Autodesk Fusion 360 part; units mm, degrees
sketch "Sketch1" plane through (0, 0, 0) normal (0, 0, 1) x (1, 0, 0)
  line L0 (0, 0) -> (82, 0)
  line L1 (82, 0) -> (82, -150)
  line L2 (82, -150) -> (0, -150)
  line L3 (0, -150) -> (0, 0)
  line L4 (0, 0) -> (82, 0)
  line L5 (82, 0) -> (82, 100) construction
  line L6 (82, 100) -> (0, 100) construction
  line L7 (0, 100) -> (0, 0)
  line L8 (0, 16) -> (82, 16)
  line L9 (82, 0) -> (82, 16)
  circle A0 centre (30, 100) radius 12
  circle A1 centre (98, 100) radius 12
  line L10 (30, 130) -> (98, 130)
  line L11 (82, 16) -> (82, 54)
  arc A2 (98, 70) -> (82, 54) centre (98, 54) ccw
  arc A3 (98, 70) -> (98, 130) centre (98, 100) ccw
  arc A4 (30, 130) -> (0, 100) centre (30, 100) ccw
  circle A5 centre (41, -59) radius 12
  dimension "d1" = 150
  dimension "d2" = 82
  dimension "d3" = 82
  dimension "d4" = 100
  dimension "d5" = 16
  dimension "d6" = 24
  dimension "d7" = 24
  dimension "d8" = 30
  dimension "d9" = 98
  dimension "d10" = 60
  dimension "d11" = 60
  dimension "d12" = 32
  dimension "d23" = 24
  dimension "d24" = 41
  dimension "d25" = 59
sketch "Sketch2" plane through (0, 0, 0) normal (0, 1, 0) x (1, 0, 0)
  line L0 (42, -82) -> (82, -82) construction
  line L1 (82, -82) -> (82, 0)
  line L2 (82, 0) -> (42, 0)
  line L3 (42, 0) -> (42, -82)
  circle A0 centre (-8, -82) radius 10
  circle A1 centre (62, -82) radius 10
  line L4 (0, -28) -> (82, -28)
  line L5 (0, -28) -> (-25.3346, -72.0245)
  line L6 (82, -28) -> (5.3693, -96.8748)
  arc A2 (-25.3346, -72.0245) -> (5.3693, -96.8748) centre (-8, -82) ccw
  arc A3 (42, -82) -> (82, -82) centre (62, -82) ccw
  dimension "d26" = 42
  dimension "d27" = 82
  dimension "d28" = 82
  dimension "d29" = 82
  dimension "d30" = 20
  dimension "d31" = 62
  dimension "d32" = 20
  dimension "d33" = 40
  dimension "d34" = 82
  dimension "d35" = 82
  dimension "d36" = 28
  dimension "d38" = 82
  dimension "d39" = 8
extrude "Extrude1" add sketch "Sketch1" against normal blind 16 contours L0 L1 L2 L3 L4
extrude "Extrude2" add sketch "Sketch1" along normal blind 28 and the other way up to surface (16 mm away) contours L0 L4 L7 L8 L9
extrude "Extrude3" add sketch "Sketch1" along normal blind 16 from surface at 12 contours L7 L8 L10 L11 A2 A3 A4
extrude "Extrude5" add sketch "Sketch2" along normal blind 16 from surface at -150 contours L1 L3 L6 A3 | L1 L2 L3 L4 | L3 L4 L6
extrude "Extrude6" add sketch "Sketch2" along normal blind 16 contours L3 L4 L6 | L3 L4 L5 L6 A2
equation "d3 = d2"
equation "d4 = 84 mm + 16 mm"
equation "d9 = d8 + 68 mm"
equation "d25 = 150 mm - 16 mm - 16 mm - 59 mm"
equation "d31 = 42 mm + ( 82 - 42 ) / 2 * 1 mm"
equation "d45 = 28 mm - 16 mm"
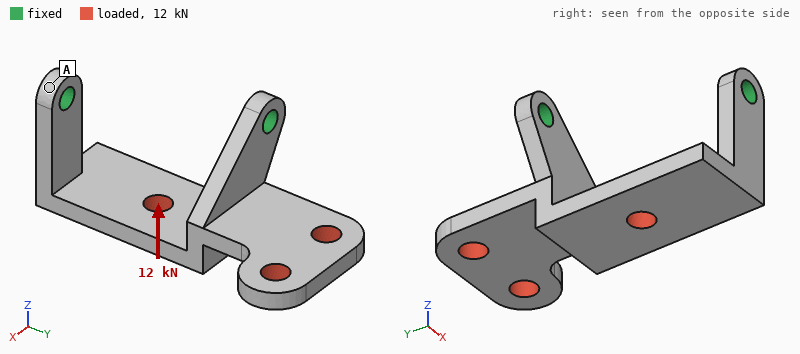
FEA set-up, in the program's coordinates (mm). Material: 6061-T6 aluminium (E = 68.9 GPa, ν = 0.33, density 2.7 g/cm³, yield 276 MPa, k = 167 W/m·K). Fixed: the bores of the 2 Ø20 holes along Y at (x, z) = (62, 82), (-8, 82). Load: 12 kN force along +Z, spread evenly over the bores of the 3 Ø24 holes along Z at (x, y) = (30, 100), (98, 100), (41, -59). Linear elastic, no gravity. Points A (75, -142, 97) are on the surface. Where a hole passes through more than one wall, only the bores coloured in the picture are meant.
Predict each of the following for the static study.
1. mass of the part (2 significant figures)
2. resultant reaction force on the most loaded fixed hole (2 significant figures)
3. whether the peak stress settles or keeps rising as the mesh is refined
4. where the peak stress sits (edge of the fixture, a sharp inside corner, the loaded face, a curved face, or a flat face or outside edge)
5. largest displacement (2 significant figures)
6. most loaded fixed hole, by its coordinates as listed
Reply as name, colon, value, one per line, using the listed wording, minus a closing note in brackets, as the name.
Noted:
mass of the part: 1.5 kg
resultant reaction force on the most loaded fixed hole: 14 kN
whether the peak stress settles or keeps rising as the mesh is refined: keeps rising
where the peak stress sits: edge of the fixture
largest displacement: 3.4 mm
most loaded fixed hole, by its coordinates as listed: (-8, 82)
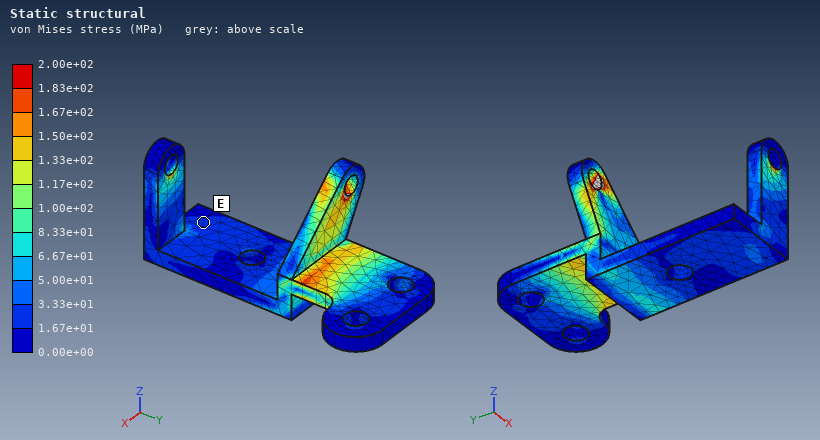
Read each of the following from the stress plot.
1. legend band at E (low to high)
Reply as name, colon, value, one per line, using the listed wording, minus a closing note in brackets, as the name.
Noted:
legend band at E: 1.67e+01 to 3.33e+01 MPa
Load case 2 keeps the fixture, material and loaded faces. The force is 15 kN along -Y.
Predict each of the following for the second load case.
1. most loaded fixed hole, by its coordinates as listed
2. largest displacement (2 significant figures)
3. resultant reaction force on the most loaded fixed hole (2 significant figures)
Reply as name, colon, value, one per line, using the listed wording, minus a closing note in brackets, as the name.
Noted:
most loaded fixed hole, by its coordinates as listed: (-8, 82)
largest displacement: 0.90 mm
resultant reaction force on the most loaded fixed hole: 9.4 kN
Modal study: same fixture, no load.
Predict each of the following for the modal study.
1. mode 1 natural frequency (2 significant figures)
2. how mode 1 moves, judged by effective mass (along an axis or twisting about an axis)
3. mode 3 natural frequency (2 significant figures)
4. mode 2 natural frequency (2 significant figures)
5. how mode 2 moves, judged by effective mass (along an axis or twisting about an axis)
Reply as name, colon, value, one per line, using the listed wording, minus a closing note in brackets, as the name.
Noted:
mode 1 natural frequency: 510 Hz
how mode 1 moves, judged by effective mass: along Z
mode 3 natural frequency: 1100 Hz
mode 2 natural frequency: 740 Hz
how mode 2 moves, judged by effective mass: along Y
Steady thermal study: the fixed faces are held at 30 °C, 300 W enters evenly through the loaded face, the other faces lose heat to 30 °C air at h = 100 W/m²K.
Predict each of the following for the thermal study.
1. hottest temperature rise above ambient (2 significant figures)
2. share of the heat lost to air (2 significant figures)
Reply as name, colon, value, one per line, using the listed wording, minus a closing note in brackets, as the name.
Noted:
hottest temperature rise above ambient: 70 K
share of the heat lost to air: 78 %
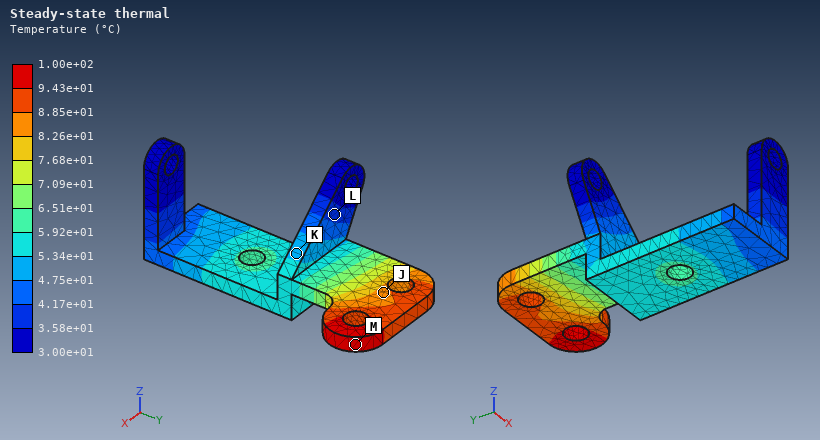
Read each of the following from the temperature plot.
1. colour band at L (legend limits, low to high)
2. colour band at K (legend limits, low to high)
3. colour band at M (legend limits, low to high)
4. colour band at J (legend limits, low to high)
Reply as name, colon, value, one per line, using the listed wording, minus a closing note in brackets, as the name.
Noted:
colour band at L: 3.58e+01 to 4.17e+01 °C
colour band at K: 4.75e+01 to 5.34e+01 °C
colour band at M: 9.43e+01 to 1.00e+02 °C
colour band at J: 8.26e+01 to 8.85e+01 °C
